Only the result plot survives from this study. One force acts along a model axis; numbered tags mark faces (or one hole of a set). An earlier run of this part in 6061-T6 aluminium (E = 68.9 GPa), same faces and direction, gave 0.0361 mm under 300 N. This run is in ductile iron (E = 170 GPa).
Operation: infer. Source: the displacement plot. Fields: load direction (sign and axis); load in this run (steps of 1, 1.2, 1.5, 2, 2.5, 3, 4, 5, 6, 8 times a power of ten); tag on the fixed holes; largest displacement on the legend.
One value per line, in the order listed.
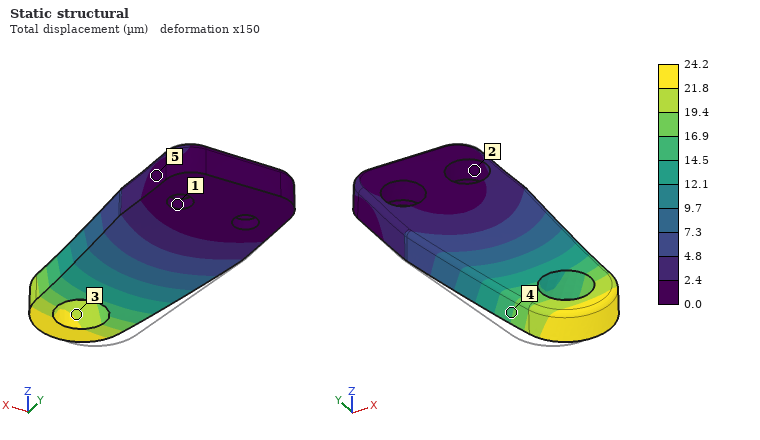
+X
500 N
1
24.2 µm
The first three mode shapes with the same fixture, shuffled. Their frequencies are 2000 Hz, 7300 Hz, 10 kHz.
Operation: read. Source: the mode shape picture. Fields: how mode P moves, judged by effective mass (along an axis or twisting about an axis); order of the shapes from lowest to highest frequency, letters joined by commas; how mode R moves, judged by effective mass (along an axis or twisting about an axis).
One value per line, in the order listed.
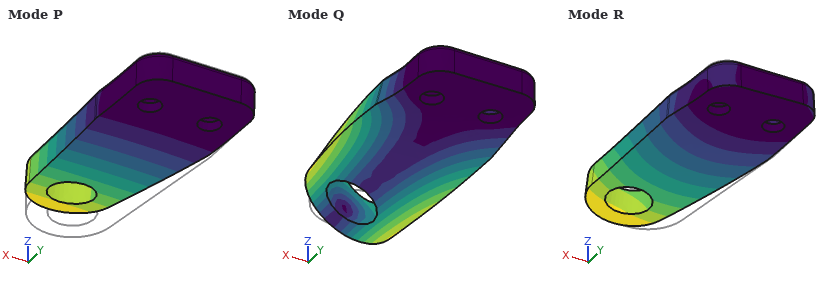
along Z
P, R, Q
along X
